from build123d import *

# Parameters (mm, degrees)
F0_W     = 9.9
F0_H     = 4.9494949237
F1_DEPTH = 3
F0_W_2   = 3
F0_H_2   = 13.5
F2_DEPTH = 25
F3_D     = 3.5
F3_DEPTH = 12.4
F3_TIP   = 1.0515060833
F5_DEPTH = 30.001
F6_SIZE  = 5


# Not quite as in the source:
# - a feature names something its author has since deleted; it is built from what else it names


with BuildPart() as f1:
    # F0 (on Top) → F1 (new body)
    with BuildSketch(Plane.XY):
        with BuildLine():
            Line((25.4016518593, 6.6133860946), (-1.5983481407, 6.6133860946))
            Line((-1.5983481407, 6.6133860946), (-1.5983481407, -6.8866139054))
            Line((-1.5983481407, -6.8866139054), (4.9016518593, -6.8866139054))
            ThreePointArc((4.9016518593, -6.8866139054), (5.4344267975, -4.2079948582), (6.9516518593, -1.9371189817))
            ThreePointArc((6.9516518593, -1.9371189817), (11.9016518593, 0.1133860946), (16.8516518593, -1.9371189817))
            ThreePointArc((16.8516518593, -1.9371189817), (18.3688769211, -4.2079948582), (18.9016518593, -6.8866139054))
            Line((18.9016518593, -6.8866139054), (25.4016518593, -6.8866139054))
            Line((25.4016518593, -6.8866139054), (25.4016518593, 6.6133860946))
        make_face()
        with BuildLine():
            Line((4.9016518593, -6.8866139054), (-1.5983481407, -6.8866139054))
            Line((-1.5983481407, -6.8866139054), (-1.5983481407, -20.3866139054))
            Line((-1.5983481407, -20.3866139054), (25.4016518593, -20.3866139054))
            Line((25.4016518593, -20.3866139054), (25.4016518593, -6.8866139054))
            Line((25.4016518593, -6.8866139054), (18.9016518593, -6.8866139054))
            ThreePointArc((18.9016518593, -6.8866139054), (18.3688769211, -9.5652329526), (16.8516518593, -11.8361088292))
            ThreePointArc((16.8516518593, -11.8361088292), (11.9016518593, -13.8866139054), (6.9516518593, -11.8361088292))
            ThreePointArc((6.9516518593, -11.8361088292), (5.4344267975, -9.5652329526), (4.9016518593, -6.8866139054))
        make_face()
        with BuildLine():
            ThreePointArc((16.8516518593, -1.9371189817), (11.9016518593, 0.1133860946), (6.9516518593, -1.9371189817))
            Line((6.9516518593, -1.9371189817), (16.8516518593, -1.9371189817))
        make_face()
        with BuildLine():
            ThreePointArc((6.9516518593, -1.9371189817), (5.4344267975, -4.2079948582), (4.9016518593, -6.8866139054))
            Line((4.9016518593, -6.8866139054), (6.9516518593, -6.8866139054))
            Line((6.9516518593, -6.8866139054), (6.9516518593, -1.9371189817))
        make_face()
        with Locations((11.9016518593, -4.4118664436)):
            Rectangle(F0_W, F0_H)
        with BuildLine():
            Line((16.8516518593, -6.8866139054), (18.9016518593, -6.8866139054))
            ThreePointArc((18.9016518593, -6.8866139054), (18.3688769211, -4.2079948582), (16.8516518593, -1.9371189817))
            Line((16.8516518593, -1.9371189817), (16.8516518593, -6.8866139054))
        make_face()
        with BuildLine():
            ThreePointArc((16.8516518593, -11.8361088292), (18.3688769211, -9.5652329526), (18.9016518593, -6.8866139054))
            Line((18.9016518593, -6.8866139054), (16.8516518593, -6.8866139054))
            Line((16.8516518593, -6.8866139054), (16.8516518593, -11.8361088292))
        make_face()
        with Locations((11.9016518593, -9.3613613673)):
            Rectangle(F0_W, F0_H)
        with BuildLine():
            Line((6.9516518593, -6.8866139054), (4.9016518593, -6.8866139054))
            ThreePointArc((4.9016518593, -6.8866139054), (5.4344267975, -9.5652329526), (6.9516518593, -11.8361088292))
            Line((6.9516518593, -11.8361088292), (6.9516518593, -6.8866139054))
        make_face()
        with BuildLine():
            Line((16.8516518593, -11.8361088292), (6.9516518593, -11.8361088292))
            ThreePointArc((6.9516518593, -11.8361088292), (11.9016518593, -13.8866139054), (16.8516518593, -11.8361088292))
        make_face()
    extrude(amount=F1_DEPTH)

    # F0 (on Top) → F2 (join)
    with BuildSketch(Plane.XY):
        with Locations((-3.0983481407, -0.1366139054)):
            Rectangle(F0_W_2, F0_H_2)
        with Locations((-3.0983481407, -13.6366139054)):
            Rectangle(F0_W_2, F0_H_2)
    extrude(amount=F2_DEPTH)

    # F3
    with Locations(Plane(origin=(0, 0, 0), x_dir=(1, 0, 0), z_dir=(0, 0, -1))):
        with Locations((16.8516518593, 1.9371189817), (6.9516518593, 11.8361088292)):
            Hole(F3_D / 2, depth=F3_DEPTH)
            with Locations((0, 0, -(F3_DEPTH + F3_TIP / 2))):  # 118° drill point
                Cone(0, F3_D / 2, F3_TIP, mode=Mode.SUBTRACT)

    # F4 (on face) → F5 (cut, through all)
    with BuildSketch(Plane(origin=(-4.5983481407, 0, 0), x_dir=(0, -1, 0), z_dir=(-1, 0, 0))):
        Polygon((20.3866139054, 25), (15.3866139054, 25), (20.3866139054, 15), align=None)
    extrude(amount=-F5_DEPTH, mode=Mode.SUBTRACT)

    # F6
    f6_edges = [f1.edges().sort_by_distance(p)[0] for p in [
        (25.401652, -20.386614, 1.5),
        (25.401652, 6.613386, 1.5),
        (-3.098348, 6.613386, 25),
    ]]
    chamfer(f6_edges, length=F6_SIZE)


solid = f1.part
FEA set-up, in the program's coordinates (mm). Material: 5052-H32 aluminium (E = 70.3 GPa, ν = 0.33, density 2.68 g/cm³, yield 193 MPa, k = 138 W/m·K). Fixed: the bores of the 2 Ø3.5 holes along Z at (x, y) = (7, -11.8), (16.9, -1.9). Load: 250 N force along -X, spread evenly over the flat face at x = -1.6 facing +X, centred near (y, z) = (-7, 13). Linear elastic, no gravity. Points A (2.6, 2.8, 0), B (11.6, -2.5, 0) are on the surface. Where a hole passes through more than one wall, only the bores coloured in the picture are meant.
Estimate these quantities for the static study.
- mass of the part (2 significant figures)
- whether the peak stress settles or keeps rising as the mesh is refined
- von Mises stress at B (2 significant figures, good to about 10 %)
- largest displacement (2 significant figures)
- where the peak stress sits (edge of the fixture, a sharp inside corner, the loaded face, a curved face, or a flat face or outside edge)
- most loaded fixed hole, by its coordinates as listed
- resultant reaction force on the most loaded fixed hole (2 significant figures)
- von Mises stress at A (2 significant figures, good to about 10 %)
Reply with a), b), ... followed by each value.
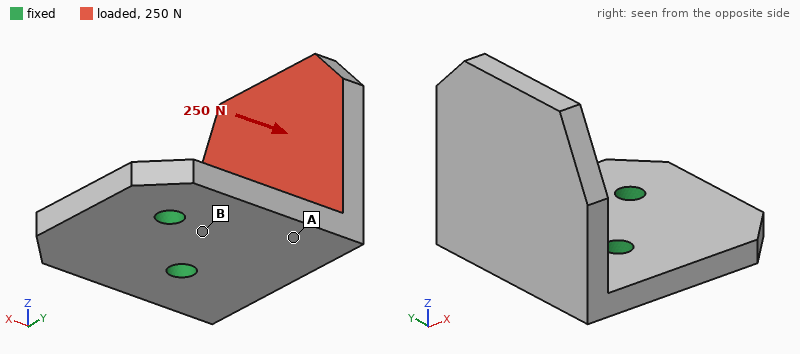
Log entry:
a) 11 g
b) keeps rising
c) 17 MPa
d) 0.26 mm
e) edge of the fixture
f) (7, -11.8)
g) 170 N
h) 54 MPa
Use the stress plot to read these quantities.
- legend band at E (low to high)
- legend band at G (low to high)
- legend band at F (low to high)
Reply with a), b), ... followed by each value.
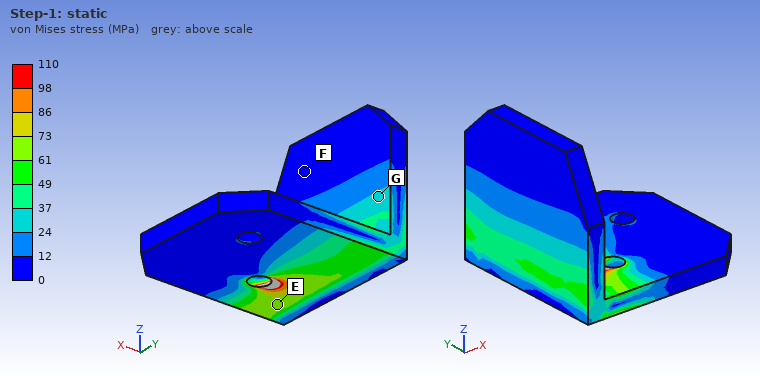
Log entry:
a) 61 to 73 MPa
b) 24 to 37 MPa
c) 0 to 12 MPa
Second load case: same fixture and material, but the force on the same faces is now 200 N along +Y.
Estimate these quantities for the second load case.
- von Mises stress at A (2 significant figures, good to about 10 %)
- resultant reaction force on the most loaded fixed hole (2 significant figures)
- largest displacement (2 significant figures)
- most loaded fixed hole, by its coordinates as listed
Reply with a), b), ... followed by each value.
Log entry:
a) 18 MPa
b) 260 N
c) 91 µm
d) (7, -11.8)
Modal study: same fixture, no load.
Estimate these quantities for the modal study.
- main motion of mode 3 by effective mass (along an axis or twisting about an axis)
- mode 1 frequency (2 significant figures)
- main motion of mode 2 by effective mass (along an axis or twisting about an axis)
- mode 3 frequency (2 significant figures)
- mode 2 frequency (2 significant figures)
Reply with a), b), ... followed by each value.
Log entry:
a) along Z
b) 2800 Hz
c) along Y
d) 9000 Hz
e) 4200 Hz
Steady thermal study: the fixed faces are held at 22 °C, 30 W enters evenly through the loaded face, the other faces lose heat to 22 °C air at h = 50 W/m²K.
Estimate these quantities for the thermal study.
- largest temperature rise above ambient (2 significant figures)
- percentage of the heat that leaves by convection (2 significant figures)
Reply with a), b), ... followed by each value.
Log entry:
a) 59 K
b) 9.4 %
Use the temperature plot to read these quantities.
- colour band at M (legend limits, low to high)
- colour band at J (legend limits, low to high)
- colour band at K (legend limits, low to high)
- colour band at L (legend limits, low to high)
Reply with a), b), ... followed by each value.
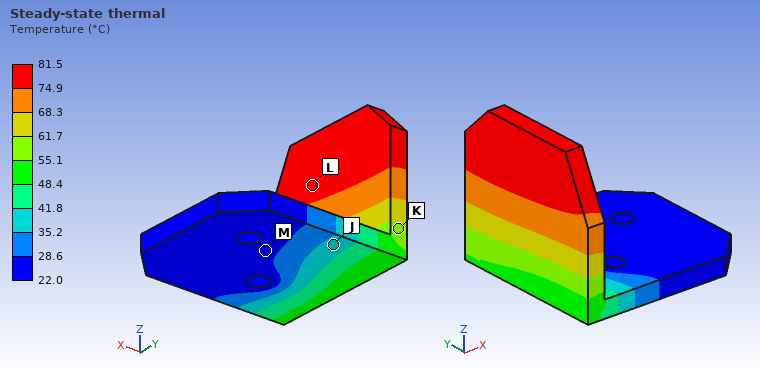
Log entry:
a) 22.0 to 28.6 °C
b) 35.2 to 41.8 °C
c) 55.1 to 61.7 °C
d) 74.9 to 81.5 °C
